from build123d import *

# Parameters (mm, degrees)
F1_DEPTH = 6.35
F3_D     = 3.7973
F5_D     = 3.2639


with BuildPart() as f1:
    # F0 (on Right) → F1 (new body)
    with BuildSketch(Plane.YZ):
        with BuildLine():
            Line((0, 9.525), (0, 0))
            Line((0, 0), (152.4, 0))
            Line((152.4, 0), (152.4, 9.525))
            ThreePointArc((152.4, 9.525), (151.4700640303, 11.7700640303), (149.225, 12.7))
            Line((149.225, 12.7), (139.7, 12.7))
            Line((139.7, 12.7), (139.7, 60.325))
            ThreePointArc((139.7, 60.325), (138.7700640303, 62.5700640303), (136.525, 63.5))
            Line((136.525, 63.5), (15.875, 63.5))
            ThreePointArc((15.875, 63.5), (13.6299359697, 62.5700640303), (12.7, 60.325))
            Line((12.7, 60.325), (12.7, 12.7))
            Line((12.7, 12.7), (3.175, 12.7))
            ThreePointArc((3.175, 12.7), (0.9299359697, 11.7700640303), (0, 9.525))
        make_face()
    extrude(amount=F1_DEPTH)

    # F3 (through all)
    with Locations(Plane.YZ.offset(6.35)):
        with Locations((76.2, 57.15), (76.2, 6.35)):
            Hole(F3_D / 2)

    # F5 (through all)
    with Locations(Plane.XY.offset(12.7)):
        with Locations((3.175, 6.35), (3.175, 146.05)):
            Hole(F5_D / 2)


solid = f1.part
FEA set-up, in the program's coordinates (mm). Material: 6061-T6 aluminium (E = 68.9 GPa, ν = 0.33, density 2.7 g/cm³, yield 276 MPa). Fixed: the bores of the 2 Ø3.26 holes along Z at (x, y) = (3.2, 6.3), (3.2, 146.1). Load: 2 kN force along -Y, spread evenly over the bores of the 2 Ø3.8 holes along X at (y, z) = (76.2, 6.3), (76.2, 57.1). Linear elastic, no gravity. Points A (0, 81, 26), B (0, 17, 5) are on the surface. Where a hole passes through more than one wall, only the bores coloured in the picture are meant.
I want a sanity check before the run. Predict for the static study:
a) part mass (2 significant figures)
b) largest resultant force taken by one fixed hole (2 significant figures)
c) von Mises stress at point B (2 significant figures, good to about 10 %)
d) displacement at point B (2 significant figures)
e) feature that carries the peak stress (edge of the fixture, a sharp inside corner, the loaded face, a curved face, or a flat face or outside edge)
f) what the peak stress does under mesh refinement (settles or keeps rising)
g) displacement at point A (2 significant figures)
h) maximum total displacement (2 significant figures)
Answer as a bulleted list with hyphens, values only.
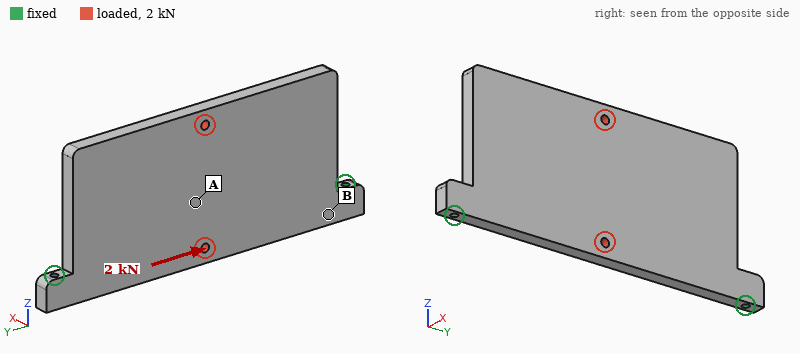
- 140 g
- 1.1 kN
- 8.7 MPa
- 2.0 µm
- edge of the fixture
- keeps rising
- 5.9 µm
- 9.6 µm
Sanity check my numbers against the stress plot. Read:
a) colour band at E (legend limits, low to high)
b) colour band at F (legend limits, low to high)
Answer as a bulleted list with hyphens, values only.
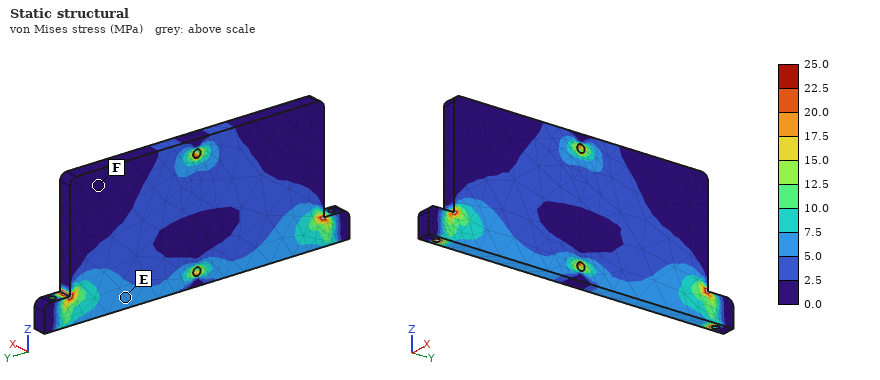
- 5.0 to 7.5 MPa
- 0.0 to 2.5 MPa
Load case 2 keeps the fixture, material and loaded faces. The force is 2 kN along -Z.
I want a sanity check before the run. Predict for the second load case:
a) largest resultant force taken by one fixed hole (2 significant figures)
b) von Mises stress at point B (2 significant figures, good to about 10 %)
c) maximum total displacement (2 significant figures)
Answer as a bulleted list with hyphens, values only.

- 1.3 kN
- 11 MPa
- 21 µm
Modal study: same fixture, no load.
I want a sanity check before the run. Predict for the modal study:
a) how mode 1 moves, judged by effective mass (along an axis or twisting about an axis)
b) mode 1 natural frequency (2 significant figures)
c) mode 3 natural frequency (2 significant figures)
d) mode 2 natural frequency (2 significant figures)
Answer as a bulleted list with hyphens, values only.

- along X
- 630 Hz
- 1800 Hz
- 1700 Hz
